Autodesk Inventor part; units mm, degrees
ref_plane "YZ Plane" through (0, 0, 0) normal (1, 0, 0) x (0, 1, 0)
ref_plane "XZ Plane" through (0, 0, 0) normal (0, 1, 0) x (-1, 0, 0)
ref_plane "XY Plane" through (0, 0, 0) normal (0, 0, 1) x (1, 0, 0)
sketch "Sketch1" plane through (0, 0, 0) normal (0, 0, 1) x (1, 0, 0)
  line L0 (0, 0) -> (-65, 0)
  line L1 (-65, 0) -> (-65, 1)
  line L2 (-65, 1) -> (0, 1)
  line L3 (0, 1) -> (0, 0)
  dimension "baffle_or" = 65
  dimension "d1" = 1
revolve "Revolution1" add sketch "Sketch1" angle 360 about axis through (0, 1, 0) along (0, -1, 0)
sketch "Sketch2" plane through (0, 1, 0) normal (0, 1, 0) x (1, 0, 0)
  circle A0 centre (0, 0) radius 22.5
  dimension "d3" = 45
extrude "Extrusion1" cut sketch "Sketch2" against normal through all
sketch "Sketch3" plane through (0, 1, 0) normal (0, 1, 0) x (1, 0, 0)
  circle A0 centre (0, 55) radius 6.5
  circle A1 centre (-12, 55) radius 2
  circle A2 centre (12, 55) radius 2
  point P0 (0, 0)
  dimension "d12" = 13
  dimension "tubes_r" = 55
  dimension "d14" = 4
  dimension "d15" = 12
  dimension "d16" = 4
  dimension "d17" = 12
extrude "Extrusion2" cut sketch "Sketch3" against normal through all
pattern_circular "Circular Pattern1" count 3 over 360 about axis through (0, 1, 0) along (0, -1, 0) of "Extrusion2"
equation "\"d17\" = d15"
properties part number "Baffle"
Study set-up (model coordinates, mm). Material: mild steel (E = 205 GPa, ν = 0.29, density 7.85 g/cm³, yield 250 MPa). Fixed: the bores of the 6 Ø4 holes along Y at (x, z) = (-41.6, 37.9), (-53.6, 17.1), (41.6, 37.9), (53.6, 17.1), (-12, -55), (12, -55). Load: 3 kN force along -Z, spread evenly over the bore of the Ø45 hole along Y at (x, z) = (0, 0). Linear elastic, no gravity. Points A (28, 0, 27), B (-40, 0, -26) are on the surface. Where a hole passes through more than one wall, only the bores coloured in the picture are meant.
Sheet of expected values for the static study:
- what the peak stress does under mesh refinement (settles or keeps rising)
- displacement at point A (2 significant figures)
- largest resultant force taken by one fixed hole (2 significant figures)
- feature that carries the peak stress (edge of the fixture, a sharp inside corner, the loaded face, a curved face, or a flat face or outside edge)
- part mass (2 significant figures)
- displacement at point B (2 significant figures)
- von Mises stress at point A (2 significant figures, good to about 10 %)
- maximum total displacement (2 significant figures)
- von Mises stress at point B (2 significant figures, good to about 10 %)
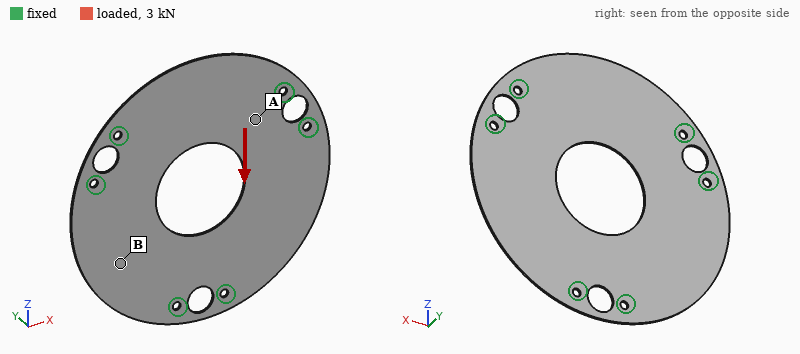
keeps rising
4.9 µm
600 N
edge of the fixture
88 g
4.5 µm
27 MPa
9.9 µm
9.1 MPa
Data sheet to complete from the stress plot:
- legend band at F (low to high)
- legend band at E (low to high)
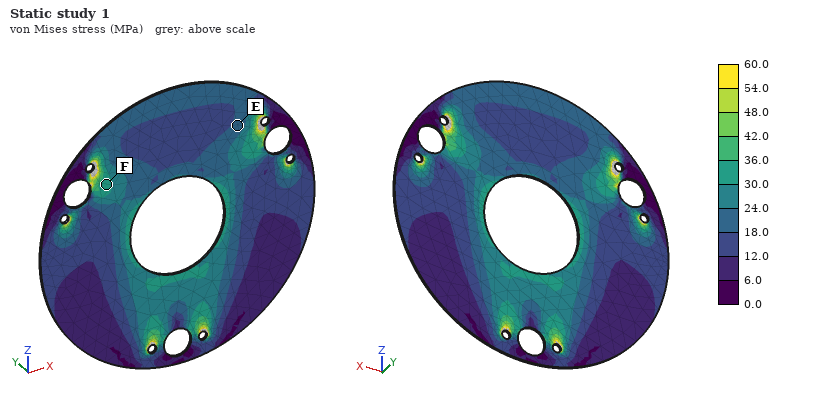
30.0 to 36.0 MPa
18.0 to 24.0 MPa
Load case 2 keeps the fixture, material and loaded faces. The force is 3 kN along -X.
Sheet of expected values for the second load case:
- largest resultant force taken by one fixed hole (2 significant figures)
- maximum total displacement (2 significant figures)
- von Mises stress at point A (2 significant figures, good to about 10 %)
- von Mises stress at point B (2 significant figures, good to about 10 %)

610 N
9.1 µm
21 MPa
14 MPa
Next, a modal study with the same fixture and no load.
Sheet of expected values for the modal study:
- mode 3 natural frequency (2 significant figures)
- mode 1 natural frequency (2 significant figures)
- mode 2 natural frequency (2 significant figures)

630 Hz
630 Hz
630 Hz
